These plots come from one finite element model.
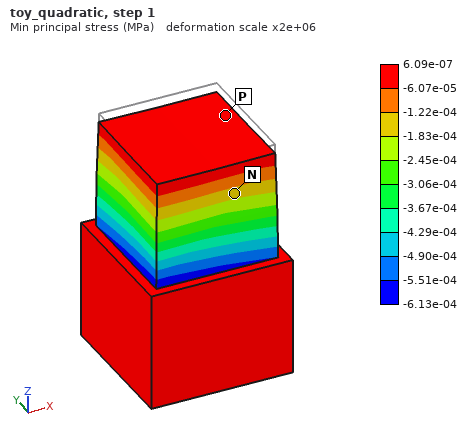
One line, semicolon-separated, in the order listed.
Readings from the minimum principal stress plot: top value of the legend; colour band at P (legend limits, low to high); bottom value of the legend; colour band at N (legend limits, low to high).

6.09e-07 MPa; -6.07e-05 to 6.09e-07 MPa; -6.13e-04 MPa; -1.83e-04 to -1.22e-04 MPa
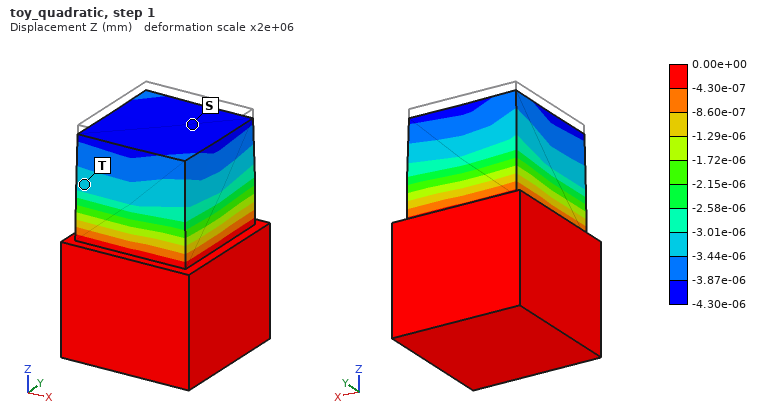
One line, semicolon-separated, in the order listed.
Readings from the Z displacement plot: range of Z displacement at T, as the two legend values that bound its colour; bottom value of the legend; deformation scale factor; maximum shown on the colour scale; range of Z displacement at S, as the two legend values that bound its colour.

-3.44e-06 to -3.01e-06 mm; -4.30e-06 mm; 2e+06; 0.00e+00 mm; -4.30e-06 to -3.87e-06 mm
